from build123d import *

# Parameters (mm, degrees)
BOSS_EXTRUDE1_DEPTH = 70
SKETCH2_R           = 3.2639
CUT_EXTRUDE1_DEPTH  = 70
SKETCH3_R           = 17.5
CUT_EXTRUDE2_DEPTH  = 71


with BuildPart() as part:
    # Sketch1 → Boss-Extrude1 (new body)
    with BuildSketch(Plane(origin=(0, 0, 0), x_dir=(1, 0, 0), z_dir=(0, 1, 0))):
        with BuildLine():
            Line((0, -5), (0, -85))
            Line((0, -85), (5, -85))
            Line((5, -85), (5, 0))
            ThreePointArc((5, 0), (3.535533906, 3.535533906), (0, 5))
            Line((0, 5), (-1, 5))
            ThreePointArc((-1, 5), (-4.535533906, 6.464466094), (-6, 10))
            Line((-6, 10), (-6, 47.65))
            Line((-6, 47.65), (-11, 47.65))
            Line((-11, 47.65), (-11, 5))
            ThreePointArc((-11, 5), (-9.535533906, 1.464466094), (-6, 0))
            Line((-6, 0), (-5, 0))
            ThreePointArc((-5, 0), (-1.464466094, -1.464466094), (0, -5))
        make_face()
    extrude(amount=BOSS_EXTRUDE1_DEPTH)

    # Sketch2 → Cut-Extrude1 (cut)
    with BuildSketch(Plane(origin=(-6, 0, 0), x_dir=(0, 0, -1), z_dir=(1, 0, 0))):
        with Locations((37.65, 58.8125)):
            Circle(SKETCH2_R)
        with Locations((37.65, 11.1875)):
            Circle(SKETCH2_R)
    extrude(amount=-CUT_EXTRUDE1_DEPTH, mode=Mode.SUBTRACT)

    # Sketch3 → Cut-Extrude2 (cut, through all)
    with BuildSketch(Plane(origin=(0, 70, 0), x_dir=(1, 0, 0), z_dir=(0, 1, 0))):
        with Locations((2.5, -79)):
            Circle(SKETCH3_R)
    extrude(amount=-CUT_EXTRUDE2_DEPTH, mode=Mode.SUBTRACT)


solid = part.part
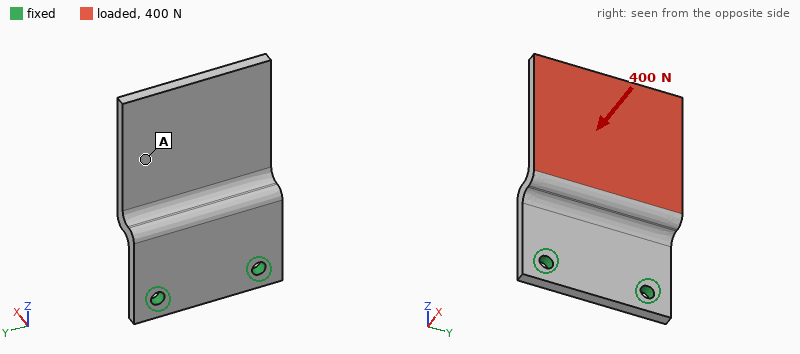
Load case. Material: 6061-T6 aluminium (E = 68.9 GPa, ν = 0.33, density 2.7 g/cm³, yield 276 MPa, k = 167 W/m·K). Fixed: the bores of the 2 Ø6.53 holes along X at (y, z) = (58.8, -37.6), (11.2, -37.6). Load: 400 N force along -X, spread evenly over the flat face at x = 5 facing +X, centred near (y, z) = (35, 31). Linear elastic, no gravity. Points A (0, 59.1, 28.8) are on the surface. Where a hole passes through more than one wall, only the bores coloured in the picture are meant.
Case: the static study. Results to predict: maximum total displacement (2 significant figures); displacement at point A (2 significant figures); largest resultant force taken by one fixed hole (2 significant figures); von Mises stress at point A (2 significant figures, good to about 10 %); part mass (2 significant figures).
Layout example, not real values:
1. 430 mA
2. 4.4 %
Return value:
1. 1.4 mm
2. 0.80 mm
3. 220 N
4. 12 MPa
5. 110 g
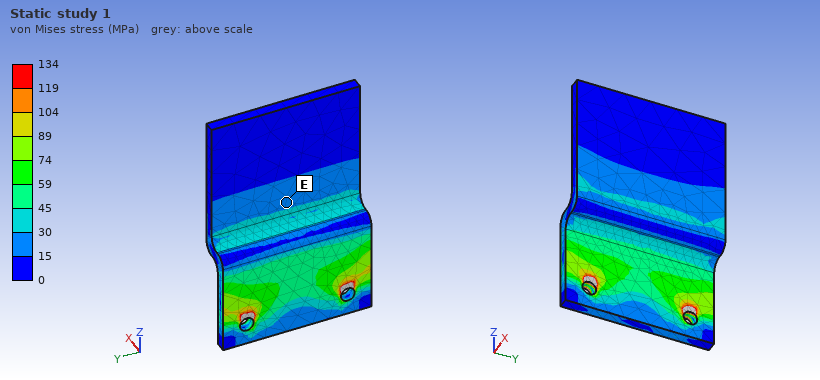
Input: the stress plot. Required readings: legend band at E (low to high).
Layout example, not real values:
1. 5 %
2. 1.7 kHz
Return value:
1. 15 to 30 MPa
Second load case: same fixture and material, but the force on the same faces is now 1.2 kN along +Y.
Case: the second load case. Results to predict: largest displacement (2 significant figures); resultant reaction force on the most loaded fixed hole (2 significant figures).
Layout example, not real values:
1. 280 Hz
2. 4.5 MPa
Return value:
1. 86 µm
2. 1.7 kN
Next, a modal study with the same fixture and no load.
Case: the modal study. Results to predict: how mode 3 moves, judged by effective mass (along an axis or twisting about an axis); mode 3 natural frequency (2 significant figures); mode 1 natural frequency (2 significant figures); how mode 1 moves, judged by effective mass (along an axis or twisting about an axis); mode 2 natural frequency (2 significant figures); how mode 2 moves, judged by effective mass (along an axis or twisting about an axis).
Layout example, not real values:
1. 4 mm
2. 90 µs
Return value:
1. along X
2. 2400 Hz
3. 410 Hz
4. along X
5. 1400 Hz
6. twisting about Z
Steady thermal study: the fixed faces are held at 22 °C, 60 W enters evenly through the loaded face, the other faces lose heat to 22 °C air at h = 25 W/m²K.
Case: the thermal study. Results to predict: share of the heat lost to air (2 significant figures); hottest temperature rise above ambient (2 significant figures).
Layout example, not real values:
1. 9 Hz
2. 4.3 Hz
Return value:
1. 19 %
2. 65 K
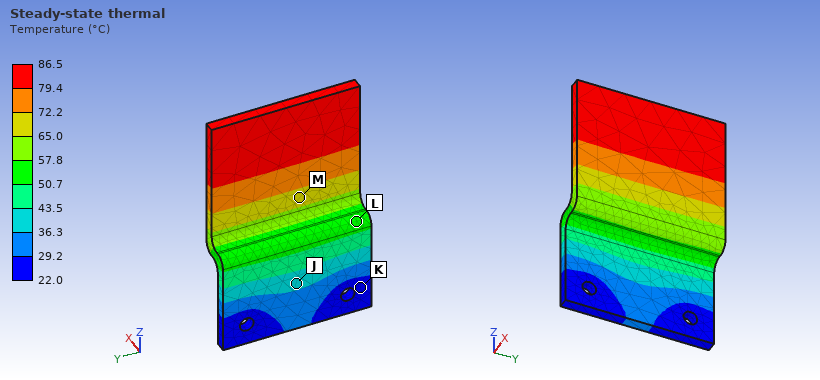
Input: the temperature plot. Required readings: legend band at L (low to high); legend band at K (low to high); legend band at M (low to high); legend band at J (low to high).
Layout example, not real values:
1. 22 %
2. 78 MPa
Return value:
1. 50.7 to 57.8 °C
2. 22.0 to 29.2 °C
3. 65.0 to 72.2 °C
4. 36.3 to 43.5 °C
